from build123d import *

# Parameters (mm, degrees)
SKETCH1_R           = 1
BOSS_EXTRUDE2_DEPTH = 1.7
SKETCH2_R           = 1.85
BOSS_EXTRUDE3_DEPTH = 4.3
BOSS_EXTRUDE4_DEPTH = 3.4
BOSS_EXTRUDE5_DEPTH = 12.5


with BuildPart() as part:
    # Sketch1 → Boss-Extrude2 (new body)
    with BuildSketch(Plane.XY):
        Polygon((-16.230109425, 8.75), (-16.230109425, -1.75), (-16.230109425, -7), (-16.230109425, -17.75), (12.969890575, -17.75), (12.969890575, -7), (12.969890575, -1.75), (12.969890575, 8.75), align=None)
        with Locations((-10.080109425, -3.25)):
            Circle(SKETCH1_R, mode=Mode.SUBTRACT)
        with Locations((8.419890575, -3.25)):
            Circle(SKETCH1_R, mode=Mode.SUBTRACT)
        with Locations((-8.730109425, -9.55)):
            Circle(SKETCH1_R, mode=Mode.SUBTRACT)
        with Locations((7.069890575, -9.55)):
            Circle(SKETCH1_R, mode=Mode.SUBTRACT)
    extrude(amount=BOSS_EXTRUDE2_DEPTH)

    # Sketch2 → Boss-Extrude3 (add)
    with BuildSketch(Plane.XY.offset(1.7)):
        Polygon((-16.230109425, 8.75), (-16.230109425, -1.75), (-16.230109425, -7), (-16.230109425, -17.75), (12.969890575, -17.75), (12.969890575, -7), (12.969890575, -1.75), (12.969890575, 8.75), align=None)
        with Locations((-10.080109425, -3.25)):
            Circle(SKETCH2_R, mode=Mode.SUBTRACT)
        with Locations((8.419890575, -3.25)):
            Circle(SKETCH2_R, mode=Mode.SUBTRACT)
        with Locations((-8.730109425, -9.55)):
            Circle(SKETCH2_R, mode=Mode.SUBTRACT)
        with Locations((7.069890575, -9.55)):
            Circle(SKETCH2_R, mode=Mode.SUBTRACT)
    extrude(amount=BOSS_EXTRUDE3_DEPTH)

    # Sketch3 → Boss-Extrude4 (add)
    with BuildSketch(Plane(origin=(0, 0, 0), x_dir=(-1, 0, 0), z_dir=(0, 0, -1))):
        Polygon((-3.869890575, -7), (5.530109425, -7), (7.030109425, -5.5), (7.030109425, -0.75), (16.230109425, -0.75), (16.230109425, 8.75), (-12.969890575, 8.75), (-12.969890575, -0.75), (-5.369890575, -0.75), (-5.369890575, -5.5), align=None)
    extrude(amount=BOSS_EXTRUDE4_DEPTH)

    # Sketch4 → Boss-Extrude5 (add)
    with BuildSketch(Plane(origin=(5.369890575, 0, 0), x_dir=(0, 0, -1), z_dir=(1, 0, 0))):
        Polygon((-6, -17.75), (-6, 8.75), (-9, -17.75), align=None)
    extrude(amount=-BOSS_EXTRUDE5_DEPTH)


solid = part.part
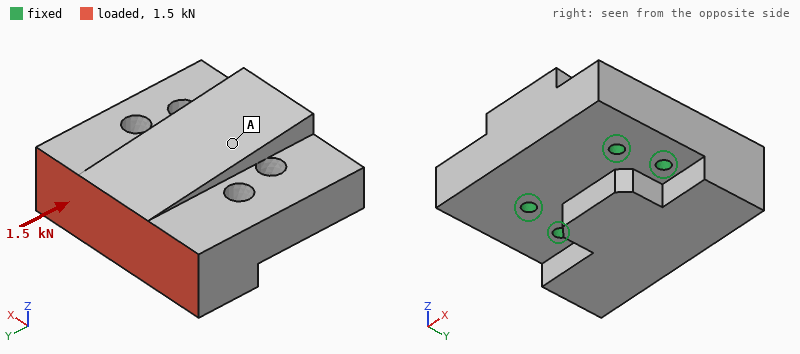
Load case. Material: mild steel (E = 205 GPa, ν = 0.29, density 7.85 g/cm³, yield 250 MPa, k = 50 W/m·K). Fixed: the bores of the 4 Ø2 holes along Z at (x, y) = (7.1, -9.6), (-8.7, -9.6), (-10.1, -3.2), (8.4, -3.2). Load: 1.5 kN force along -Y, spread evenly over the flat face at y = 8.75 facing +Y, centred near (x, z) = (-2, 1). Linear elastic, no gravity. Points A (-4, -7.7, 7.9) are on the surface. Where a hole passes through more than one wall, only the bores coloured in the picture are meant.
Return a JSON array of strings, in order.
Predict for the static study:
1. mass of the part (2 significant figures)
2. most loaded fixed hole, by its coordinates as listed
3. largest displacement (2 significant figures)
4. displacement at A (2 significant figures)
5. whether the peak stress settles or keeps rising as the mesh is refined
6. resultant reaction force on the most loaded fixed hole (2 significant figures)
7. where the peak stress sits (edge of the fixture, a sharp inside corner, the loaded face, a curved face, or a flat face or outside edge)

["48 g", "(-10.1, -3.2)", "1.1 µm", "0.65 µm", "keeps rising", "520 N", "edge of the fixture"]
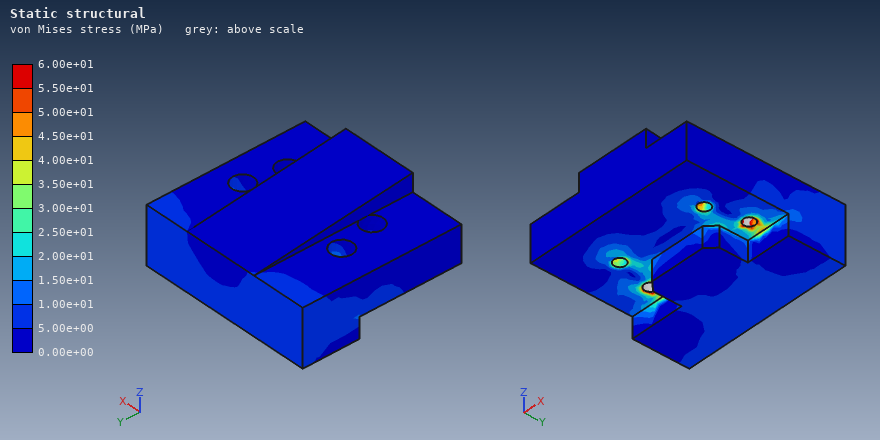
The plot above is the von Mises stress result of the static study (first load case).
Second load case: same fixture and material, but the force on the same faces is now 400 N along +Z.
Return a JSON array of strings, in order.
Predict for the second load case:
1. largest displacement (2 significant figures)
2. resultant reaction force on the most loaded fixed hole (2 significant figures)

["6.2 µm", "510 N"]
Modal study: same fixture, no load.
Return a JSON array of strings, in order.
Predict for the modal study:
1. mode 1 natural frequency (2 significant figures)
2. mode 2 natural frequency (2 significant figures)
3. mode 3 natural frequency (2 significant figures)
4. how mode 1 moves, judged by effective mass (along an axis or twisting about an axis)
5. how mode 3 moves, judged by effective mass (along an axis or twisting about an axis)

["12 kHz", "26 kHz", "27 kHz", "along Z", "along Z"]
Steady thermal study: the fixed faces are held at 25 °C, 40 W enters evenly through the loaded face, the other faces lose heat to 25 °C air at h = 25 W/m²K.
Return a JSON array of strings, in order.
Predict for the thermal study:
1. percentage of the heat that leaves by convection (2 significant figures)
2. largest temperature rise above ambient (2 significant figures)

["4.5 %", "64 K"]
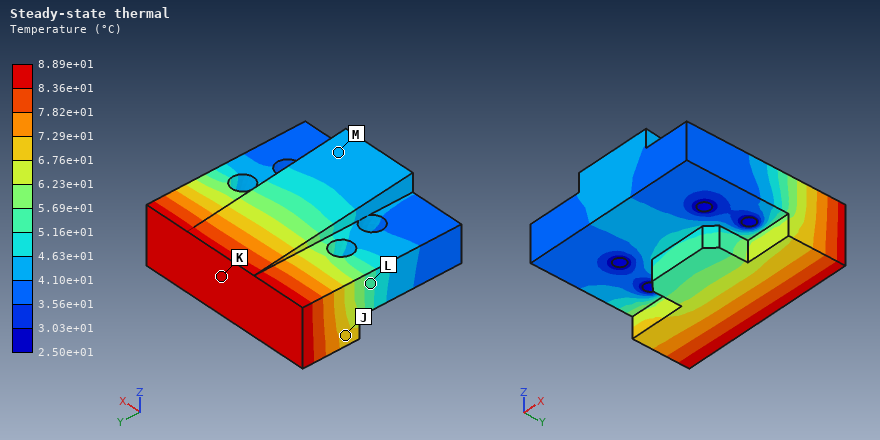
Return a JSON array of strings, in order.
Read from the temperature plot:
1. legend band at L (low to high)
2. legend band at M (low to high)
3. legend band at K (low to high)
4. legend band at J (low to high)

["5.16e+01 to 5.69e+01 °C", "4.10e+01 to 4.63e+01 °C", "8.36e+01 to 8.89e+01 °C", "6.76e+01 to 7.29e+01 °C"]
